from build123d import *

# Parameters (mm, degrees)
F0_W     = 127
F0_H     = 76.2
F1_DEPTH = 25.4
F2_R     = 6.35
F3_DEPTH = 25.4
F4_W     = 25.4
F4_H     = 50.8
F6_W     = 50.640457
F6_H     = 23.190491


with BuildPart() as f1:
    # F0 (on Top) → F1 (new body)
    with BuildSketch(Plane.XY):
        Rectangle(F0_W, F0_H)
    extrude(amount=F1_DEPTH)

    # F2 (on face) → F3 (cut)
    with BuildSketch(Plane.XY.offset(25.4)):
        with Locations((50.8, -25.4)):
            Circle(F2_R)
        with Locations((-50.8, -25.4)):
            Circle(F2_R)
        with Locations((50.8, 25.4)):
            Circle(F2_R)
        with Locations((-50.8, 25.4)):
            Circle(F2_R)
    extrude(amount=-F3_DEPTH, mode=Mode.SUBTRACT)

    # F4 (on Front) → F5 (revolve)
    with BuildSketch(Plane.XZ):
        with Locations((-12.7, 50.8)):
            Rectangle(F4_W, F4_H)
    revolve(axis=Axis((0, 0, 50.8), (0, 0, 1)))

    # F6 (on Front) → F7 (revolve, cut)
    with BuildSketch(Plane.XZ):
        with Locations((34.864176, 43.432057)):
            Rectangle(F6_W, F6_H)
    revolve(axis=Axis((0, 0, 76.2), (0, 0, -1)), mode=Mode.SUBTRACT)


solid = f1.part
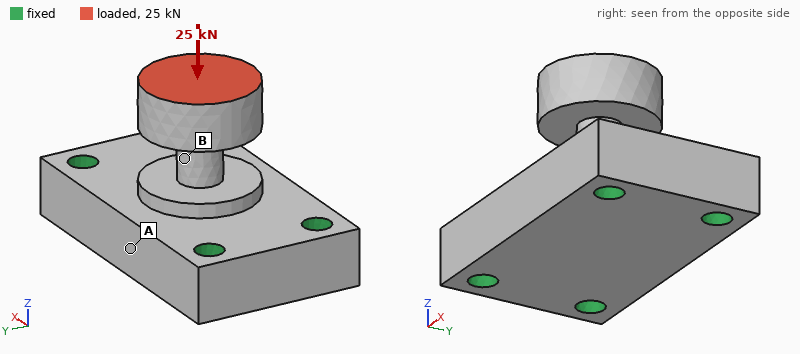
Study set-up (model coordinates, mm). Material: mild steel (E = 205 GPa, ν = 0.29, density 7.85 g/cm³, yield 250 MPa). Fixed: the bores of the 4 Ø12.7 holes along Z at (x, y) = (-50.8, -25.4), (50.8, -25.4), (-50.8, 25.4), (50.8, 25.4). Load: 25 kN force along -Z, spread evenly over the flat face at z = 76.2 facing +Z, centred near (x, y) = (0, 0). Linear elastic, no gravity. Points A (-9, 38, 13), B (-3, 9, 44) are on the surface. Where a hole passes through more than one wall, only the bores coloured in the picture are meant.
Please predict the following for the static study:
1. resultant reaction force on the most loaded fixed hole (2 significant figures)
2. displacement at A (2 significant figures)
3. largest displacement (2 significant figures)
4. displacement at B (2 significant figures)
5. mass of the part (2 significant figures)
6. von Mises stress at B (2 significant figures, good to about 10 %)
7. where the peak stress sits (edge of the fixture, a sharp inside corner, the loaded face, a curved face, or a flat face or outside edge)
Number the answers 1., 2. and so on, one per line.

1. 6.4 kN
2. 6.4 µm
3. 26 µm
4. 16 µm
5. 2.3 kg
6. 85 MPa
7. a curved face
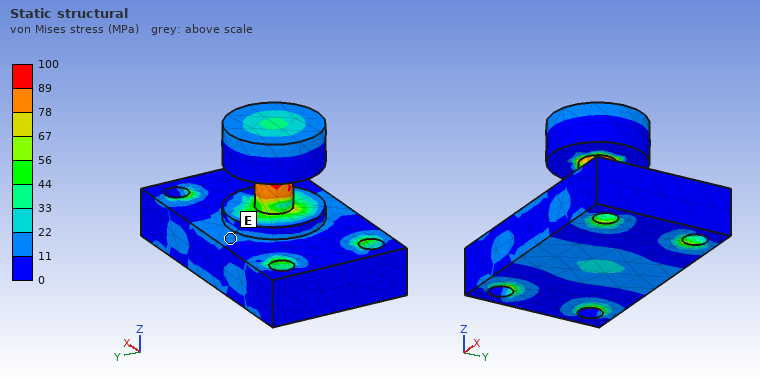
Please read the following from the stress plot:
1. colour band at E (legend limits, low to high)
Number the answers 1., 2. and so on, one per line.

1. 11 to 22 MPa
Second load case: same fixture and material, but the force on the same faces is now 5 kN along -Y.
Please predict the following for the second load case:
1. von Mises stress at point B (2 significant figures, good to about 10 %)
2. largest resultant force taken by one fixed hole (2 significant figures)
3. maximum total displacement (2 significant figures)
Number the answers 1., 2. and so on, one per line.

1. 230 MPa
2. 3.2 kN
3. 0.18 mm
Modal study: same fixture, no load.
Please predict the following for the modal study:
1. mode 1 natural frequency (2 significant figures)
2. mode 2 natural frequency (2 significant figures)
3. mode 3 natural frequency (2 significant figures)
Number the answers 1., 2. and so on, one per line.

1. 1900 Hz
2. 2000 Hz
3. 2900 Hz
